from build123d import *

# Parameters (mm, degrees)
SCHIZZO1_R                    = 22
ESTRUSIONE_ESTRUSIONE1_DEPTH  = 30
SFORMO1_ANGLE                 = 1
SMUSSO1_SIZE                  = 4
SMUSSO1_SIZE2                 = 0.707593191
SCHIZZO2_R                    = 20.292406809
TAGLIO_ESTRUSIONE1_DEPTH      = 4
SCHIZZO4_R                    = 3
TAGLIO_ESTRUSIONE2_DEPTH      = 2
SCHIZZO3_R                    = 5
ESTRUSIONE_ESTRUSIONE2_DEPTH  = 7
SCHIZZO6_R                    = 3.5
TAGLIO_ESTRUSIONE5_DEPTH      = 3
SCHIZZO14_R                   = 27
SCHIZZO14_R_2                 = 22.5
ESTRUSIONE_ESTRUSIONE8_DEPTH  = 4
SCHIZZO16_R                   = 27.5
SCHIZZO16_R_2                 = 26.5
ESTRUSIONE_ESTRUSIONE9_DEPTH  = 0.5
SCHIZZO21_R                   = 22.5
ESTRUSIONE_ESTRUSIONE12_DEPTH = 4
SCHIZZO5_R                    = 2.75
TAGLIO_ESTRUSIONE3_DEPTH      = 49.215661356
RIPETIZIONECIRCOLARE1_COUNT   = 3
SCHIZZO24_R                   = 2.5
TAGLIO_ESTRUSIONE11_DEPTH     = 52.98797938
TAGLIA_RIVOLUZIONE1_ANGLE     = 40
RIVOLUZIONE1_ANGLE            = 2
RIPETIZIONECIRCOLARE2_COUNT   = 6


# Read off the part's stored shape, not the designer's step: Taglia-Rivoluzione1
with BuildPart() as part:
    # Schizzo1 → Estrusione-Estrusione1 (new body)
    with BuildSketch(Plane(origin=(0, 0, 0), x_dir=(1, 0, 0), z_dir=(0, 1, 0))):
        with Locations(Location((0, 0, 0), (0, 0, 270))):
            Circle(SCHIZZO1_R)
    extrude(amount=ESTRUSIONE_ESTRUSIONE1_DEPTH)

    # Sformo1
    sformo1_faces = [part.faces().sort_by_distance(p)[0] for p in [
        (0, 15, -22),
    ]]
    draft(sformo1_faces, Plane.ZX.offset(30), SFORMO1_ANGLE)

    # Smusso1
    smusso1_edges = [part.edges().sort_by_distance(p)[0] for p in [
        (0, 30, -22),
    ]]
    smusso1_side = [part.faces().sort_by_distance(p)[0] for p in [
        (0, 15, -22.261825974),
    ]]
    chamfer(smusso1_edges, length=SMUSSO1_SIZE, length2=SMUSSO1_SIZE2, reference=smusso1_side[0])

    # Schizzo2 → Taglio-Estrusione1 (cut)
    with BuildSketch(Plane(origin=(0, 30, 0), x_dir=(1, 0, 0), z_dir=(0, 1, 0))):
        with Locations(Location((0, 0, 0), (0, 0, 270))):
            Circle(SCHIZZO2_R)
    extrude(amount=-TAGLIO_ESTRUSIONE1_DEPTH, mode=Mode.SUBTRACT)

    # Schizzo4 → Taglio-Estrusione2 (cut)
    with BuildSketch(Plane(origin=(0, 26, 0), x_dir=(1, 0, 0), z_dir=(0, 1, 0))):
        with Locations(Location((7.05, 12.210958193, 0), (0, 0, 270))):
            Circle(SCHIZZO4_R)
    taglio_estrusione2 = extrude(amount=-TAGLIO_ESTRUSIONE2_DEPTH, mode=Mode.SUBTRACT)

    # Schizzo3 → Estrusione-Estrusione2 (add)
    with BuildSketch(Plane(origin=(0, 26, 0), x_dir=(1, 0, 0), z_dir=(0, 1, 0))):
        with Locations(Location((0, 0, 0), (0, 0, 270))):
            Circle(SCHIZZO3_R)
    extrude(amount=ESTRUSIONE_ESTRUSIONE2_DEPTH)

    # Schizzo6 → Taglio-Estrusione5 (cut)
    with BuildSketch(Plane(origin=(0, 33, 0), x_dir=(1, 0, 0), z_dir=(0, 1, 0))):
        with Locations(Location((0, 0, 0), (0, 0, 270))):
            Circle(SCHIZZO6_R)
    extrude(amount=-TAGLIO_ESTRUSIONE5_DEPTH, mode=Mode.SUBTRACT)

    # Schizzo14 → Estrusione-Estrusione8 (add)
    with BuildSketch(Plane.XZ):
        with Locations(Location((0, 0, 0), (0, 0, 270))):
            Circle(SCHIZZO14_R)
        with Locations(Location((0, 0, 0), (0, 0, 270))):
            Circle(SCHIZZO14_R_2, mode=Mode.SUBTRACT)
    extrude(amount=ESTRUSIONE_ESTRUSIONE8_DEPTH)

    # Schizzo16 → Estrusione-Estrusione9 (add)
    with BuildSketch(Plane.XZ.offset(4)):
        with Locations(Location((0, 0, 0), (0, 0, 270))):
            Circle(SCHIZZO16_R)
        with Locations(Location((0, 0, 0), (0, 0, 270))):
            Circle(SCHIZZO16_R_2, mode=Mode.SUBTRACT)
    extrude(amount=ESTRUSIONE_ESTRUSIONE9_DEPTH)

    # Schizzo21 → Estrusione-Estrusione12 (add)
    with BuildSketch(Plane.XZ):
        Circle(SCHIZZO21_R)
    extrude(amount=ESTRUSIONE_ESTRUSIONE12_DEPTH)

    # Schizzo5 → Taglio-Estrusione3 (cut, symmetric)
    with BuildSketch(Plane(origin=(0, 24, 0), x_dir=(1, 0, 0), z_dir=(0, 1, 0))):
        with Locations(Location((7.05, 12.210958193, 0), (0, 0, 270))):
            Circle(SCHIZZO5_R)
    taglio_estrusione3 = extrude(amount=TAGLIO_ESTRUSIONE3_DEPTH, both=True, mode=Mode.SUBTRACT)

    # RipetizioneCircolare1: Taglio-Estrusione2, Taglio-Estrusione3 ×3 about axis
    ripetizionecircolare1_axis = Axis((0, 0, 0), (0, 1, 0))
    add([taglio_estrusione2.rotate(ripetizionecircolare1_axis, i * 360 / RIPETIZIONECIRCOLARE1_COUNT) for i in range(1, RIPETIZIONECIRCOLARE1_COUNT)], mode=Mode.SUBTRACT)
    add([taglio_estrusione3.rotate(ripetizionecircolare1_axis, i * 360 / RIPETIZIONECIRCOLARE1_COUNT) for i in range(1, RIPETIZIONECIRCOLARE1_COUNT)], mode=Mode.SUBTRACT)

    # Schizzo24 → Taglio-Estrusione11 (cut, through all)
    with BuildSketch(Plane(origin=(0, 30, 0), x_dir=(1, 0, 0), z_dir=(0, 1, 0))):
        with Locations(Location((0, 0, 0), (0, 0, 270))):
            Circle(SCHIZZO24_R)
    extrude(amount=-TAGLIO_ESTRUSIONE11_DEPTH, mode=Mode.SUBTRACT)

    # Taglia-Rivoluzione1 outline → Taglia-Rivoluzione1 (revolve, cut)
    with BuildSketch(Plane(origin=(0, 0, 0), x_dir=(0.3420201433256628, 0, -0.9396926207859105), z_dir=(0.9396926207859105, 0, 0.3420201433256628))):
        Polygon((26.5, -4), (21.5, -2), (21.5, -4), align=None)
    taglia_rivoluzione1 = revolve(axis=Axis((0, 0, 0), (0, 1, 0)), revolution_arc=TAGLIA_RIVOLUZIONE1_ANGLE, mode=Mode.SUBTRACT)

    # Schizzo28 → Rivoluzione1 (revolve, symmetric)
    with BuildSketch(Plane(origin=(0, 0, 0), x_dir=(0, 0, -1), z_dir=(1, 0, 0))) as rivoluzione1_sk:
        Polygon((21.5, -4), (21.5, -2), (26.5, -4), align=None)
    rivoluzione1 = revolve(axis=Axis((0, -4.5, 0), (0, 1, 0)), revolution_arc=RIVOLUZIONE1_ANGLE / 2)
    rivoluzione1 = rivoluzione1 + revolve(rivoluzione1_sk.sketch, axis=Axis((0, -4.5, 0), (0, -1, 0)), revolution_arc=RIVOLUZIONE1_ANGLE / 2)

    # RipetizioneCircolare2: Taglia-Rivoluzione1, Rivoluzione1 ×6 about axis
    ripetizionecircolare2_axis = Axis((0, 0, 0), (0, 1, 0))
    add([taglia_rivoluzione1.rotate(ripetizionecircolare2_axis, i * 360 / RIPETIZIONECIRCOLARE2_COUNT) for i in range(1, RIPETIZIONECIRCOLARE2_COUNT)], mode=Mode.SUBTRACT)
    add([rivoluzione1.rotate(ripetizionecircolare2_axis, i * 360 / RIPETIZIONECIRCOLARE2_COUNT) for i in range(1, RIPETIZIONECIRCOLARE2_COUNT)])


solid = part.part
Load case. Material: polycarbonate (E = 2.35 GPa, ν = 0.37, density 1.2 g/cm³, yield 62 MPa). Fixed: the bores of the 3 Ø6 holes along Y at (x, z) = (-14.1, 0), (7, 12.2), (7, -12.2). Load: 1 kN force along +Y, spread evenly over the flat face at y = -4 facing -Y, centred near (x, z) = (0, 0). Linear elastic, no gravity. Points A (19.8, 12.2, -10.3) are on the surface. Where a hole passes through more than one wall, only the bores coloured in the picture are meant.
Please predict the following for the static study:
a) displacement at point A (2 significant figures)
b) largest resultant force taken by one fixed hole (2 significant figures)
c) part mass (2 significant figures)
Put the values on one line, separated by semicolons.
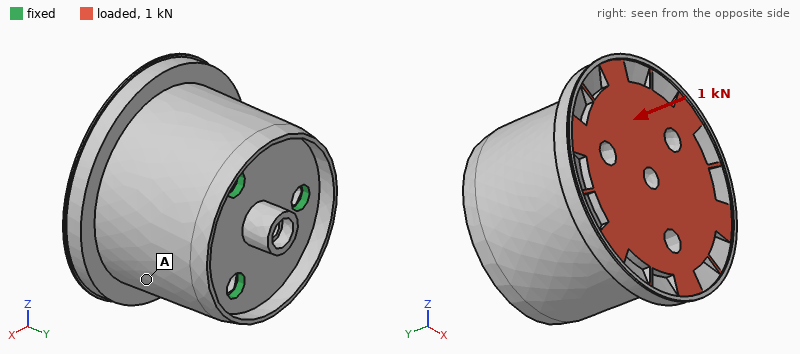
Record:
17 µm; 340 N; 57 g
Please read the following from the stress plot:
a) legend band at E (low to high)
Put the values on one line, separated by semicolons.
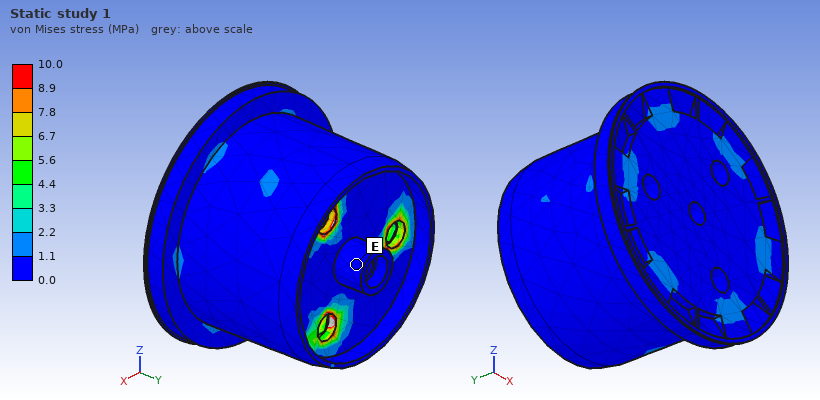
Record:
0.0 to 1.1 MPa
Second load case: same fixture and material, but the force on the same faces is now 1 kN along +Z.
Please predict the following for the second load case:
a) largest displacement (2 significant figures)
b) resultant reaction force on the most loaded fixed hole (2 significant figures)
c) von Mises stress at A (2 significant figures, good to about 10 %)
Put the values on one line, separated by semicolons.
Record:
0.23 mm; 1.1 kN; 2.4 MPa
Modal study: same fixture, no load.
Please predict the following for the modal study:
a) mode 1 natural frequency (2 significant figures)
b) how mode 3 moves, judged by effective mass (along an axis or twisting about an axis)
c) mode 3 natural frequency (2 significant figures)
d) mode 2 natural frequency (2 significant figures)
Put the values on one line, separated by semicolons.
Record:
2400 Hz; twisting about Y; 4400 Hz; 2400 Hz
